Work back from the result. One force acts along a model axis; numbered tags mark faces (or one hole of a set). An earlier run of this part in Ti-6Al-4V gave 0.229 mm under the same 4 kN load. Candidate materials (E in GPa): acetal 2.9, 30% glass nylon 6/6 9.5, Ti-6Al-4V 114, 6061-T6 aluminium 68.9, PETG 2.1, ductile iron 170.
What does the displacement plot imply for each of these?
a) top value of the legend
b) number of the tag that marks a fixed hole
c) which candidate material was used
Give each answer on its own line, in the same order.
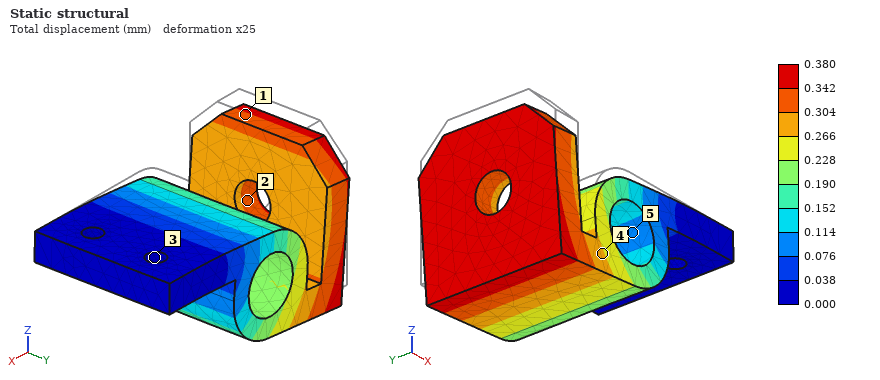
0.380 mm
3
6061-T6 aluminium
